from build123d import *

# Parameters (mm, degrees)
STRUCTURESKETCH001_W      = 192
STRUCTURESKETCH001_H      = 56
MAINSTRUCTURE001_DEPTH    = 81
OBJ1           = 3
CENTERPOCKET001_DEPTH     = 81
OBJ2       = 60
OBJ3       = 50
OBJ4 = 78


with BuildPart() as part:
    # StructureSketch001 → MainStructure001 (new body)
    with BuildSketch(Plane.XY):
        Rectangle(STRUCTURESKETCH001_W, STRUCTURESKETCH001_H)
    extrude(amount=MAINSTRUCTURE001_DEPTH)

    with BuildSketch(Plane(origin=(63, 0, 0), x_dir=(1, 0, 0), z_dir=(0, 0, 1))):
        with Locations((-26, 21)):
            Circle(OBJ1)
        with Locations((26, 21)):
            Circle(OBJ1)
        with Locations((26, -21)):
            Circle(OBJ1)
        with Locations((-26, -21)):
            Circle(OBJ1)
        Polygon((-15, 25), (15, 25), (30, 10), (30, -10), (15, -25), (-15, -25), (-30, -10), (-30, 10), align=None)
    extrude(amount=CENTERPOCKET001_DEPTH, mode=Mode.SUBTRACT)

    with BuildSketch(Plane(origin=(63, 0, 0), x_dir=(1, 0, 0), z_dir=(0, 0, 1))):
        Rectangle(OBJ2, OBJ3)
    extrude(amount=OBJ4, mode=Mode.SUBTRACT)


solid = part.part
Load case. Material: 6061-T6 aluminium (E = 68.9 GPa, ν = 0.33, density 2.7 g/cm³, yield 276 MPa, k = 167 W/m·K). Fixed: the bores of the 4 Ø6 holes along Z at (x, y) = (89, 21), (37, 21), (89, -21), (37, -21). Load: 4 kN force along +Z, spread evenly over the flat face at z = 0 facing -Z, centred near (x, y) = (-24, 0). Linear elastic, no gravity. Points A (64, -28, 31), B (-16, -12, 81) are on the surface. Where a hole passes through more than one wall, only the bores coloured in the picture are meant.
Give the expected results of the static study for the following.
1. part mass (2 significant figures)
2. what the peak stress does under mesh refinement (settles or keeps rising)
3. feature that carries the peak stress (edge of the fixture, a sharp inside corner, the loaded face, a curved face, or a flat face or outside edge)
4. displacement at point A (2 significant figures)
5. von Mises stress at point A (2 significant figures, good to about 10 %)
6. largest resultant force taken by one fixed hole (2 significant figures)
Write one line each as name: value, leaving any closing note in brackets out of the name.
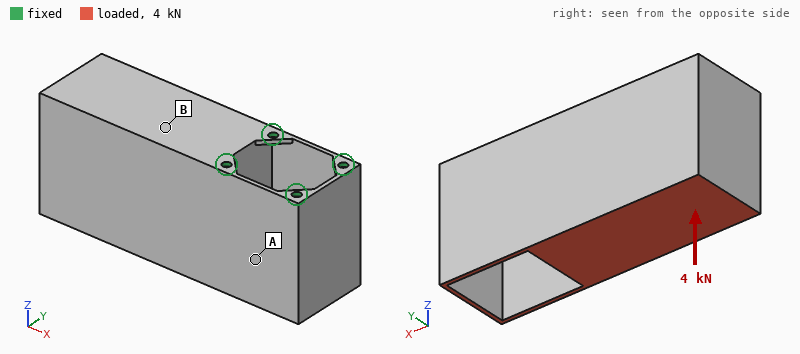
part mass: 1.7 kg
what the peak stress does under mesh refinement: keeps rising
feature that carries the peak stress: edge of the fixture
displacement at point A: 0.053 mm
von Mises stress at point A: 19 MPa
largest resultant force taken by one fixed hole: 4.2 kN
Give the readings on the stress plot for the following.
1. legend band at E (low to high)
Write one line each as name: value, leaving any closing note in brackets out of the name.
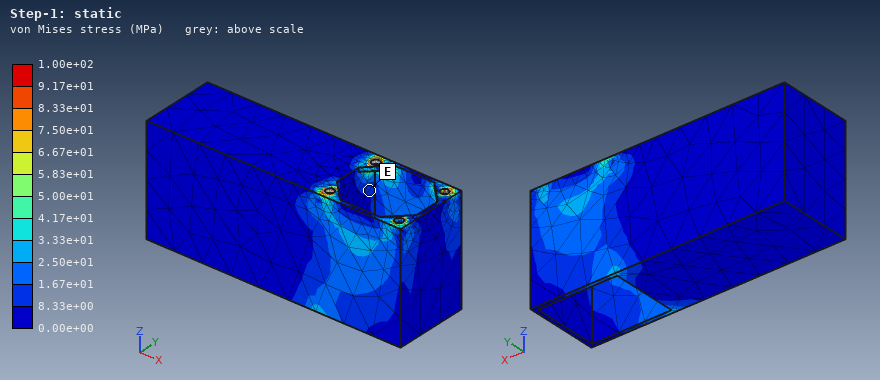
legend band at E: 8.33e+00 to 1.67e+01 MPa
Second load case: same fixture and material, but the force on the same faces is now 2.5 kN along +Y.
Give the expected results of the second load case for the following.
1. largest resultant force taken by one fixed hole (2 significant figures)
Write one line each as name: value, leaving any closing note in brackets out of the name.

largest resultant force taken by one fixed hole: 4.5 kN
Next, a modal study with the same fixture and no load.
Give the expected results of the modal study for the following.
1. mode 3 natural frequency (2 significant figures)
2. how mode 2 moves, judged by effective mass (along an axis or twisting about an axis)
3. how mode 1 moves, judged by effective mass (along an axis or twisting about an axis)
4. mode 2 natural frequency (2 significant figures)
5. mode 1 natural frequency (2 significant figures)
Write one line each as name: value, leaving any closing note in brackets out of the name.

mode 3 natural frequency: 1500 Hz
how mode 2 moves, judged by effective mass: along Y
how mode 1 moves, judged by effective mass: along Z
mode 2 natural frequency: 870 Hz
mode 1 natural frequency: 610 Hz
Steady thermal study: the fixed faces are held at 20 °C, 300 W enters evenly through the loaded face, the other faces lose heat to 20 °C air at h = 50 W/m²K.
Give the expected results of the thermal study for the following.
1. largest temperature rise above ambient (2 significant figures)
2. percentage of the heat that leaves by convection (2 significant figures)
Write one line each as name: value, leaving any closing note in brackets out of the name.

largest temperature rise above ambient: 71 K
percentage of the heat that leaves by convection: 48 %
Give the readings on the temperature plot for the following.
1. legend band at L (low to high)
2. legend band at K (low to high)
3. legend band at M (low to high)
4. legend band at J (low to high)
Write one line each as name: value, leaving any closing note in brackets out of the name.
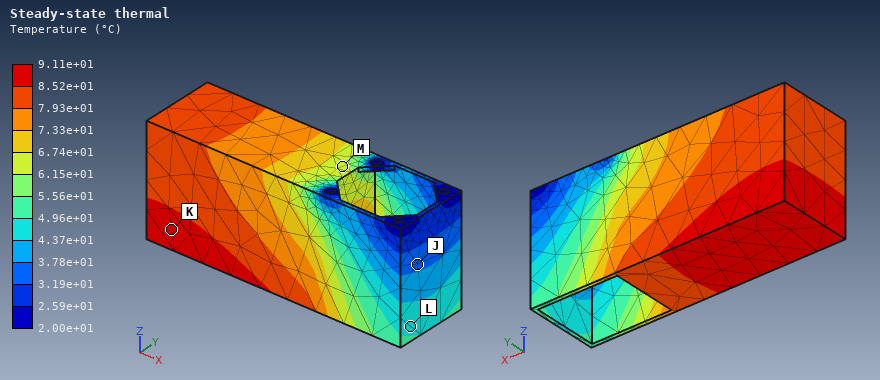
legend band at L: 4.37e+01 to 4.96e+01 °C
legend band at K: 8.52e+01 to 9.11e+01 °C
legend band at M: 6.15e+01 to 6.74e+01 °C
legend band at J: 3.19e+01 to 3.78e+01 °C
